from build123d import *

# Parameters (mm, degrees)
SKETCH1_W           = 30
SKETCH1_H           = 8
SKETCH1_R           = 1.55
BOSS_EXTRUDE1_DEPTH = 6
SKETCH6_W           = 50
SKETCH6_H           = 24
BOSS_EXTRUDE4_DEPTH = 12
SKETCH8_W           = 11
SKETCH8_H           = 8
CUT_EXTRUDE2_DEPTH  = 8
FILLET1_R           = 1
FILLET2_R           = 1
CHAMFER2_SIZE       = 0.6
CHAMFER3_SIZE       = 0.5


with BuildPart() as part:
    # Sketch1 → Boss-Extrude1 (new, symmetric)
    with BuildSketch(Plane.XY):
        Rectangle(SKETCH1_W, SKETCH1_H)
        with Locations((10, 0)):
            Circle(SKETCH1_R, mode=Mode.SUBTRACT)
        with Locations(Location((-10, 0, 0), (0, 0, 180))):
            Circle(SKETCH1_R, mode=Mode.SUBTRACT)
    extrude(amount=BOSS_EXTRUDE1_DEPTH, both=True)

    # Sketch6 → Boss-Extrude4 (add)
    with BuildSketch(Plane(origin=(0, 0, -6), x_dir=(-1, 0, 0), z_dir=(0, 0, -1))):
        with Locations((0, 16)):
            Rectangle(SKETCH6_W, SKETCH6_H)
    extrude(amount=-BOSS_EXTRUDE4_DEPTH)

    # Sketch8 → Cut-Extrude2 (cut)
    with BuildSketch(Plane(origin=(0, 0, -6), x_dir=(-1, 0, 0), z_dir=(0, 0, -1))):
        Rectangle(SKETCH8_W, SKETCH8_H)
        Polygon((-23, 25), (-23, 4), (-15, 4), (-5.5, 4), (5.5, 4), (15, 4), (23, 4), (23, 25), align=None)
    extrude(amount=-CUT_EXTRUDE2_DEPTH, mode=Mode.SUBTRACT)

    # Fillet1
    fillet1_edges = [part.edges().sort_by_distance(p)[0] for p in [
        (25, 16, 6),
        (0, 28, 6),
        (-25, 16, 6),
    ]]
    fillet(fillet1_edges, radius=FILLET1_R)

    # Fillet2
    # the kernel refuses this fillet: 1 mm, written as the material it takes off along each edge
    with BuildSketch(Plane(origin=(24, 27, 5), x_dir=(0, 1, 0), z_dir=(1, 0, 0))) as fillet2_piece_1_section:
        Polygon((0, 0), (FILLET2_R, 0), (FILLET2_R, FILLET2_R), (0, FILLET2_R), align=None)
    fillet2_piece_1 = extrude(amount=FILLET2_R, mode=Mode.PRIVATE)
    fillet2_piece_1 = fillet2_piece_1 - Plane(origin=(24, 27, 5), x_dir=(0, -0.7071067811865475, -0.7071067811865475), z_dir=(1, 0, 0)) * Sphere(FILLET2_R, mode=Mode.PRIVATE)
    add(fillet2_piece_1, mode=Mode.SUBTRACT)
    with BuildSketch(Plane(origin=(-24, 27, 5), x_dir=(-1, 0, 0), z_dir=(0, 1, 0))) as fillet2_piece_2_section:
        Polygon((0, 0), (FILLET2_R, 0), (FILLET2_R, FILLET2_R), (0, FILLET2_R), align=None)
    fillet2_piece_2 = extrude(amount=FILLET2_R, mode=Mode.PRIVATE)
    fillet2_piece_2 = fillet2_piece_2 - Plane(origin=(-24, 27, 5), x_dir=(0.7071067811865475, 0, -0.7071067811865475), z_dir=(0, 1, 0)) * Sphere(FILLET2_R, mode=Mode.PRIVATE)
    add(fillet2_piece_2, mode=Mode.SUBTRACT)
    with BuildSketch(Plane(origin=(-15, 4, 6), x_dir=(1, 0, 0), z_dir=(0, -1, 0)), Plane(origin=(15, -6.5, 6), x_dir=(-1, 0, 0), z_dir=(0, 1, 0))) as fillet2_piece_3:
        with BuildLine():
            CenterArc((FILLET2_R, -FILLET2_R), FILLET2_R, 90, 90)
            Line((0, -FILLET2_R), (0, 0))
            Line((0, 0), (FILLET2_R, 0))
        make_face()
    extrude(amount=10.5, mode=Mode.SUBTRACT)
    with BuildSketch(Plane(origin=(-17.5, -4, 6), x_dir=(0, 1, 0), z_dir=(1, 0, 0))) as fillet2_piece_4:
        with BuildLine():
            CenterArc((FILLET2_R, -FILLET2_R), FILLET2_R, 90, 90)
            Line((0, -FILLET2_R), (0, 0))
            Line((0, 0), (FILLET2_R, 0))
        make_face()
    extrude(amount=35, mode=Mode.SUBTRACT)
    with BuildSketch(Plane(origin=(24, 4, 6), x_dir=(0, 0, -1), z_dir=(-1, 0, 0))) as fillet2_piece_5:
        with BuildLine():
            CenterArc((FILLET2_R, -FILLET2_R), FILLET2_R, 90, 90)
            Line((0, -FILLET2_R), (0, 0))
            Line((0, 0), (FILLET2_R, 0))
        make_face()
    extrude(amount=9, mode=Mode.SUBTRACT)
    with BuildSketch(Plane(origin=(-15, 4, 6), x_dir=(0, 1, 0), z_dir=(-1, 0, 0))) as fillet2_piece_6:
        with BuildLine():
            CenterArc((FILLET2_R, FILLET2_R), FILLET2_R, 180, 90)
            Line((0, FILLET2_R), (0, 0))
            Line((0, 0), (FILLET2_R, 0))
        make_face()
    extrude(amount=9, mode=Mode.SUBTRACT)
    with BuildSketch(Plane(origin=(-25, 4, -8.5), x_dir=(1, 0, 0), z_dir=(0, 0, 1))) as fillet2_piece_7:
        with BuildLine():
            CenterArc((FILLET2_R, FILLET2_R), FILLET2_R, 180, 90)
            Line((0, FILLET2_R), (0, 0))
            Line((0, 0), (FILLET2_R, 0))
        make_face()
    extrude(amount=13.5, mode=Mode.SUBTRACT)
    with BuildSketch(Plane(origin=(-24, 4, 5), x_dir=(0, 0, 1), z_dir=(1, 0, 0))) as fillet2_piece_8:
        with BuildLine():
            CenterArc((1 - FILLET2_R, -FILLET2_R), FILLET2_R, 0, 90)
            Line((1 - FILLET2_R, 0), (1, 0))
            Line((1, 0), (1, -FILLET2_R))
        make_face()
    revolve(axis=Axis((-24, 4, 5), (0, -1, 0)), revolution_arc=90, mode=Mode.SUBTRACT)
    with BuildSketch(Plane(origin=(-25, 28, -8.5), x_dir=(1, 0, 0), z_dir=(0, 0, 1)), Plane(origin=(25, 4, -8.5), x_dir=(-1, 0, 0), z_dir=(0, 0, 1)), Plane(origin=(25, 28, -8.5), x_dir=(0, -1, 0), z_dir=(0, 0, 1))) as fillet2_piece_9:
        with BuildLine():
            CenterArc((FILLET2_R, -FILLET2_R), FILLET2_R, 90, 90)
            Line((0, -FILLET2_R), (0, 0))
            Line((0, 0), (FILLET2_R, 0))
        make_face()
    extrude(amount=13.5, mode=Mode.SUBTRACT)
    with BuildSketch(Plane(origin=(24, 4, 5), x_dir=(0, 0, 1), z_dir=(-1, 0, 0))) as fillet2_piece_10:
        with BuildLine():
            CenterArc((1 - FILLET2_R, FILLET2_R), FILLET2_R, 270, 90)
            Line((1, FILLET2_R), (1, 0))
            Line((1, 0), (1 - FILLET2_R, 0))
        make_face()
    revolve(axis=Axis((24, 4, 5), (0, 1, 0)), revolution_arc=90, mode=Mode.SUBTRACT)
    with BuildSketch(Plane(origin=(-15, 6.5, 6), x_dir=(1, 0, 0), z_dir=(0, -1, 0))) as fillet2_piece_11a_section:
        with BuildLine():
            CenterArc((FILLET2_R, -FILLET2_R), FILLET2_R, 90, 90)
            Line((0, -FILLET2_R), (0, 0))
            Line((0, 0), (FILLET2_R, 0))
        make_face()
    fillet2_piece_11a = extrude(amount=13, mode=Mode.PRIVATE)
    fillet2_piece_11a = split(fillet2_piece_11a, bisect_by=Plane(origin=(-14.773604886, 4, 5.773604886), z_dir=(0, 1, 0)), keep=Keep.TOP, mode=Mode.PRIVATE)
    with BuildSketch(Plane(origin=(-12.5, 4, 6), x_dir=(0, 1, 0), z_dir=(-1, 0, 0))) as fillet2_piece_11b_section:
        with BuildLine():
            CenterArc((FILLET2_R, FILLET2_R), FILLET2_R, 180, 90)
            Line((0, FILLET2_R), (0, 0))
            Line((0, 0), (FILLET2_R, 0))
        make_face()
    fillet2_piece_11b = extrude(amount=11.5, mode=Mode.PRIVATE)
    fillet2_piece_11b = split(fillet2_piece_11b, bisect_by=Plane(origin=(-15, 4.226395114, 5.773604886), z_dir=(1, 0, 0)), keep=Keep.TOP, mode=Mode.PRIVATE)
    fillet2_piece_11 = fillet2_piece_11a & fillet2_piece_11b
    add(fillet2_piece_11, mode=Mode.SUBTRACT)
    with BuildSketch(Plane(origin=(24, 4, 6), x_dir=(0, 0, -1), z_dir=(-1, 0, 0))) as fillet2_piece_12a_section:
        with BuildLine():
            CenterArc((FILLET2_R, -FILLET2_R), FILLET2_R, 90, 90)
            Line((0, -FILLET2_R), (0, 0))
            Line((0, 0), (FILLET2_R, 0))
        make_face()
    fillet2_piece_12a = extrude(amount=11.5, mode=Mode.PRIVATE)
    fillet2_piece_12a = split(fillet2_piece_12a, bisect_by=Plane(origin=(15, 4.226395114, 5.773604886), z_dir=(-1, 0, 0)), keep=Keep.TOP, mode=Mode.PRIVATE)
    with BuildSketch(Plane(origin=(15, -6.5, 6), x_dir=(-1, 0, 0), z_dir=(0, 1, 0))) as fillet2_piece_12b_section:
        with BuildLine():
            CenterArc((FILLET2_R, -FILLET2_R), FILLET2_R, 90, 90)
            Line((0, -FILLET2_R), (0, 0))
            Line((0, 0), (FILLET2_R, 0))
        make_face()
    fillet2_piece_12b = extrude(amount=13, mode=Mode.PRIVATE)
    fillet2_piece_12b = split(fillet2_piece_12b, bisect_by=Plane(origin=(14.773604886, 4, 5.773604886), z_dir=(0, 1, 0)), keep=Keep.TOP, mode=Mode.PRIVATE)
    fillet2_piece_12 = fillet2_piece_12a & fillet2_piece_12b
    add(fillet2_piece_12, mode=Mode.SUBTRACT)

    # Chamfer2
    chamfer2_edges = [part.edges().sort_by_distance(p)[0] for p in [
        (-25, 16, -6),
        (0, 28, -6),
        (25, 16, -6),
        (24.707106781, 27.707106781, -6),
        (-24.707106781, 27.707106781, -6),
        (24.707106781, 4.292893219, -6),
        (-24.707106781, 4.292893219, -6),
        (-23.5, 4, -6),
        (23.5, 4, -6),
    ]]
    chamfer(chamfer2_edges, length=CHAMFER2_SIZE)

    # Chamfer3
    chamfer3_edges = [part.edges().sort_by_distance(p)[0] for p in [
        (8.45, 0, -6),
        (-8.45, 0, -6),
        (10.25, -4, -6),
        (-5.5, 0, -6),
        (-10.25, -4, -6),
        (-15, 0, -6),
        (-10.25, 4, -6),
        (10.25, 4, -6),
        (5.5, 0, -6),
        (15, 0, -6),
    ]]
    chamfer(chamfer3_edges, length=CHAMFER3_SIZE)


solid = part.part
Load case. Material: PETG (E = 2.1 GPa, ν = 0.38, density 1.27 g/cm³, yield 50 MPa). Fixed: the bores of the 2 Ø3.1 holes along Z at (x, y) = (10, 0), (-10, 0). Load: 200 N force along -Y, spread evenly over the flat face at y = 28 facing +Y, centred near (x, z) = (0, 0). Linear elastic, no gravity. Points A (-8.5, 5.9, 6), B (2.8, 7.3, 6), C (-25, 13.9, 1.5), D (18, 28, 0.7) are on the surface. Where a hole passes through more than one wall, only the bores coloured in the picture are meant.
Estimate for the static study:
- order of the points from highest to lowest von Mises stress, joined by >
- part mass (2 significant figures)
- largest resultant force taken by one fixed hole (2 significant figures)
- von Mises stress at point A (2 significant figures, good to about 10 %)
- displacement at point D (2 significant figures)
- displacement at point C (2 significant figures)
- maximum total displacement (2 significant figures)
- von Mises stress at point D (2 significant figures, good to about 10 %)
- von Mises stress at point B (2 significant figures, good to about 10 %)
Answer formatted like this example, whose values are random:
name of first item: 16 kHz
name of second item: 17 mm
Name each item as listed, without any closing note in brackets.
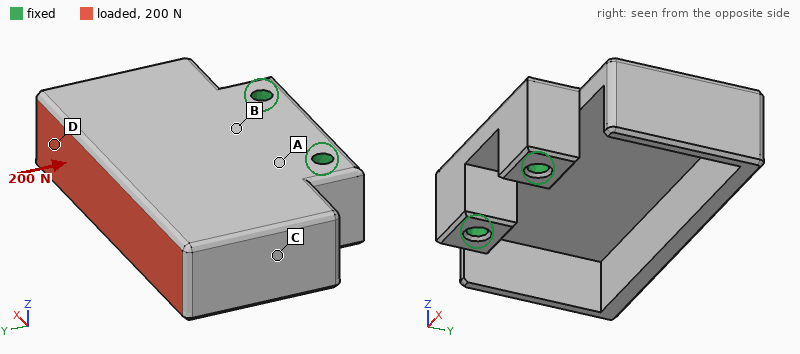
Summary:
order of the points from highest to lowest von Mises stress, joined by >: A > B > D > C
part mass: 11 g
largest resultant force taken by one fixed hole: 100 N
von Mises stress at point A: 7.0 MPa
displacement at point D: 0.58 mm
displacement at point C: 0.17 mm
maximum total displacement: 0.70 mm
von Mises stress at point D: 3.6 MPa
von Mises stress at point B: 5.8 MPa
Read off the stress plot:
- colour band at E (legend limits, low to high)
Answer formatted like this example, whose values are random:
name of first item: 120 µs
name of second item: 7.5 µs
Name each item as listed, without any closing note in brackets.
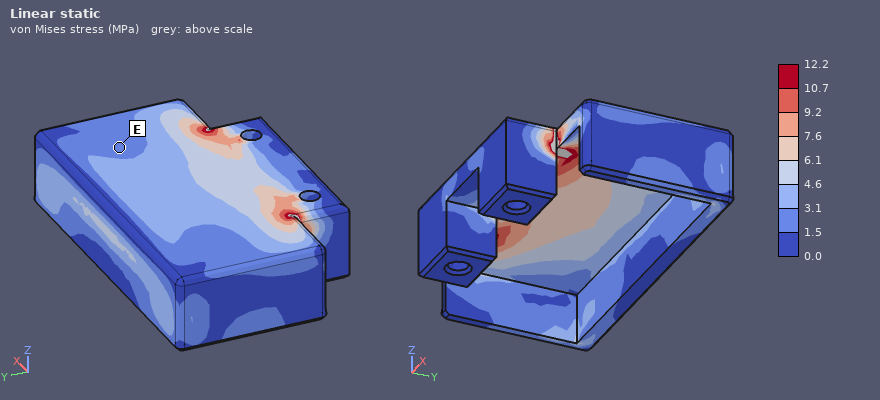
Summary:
colour band at E: 1.5 to 3.1 MPa
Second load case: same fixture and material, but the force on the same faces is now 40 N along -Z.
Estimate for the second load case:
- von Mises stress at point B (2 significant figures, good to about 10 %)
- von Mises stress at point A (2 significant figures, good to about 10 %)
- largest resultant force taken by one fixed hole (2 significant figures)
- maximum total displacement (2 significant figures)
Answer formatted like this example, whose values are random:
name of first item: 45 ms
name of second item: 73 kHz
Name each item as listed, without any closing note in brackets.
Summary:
von Mises stress at point B: 6.9 MPa
von Mises stress at point A: 9.6 MPa
largest resultant force taken by one fixed hole: 20 N
maximum total displacement: 0.62 mm
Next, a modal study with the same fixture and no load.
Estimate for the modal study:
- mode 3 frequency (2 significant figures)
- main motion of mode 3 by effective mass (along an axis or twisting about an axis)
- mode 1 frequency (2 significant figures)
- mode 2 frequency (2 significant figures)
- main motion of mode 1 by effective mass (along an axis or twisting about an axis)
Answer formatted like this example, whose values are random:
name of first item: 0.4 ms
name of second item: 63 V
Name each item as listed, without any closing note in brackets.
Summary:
mode 3 frequency: 2500 Hz
main motion of mode 3 by effective mass: along X
mode 1 frequency: 730 Hz
mode 2 frequency: 1000 Hz
main motion of mode 1 by effective mass: along Z
